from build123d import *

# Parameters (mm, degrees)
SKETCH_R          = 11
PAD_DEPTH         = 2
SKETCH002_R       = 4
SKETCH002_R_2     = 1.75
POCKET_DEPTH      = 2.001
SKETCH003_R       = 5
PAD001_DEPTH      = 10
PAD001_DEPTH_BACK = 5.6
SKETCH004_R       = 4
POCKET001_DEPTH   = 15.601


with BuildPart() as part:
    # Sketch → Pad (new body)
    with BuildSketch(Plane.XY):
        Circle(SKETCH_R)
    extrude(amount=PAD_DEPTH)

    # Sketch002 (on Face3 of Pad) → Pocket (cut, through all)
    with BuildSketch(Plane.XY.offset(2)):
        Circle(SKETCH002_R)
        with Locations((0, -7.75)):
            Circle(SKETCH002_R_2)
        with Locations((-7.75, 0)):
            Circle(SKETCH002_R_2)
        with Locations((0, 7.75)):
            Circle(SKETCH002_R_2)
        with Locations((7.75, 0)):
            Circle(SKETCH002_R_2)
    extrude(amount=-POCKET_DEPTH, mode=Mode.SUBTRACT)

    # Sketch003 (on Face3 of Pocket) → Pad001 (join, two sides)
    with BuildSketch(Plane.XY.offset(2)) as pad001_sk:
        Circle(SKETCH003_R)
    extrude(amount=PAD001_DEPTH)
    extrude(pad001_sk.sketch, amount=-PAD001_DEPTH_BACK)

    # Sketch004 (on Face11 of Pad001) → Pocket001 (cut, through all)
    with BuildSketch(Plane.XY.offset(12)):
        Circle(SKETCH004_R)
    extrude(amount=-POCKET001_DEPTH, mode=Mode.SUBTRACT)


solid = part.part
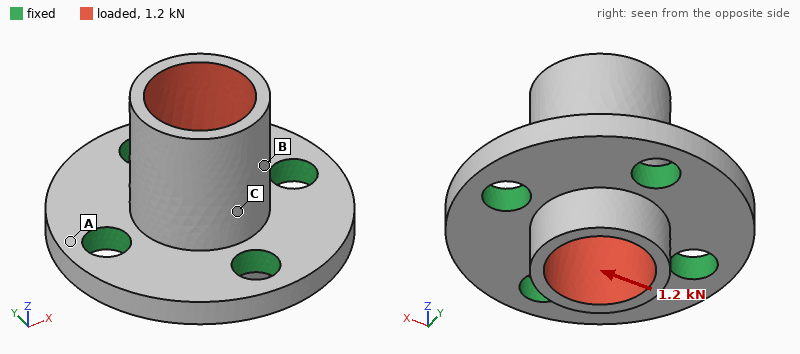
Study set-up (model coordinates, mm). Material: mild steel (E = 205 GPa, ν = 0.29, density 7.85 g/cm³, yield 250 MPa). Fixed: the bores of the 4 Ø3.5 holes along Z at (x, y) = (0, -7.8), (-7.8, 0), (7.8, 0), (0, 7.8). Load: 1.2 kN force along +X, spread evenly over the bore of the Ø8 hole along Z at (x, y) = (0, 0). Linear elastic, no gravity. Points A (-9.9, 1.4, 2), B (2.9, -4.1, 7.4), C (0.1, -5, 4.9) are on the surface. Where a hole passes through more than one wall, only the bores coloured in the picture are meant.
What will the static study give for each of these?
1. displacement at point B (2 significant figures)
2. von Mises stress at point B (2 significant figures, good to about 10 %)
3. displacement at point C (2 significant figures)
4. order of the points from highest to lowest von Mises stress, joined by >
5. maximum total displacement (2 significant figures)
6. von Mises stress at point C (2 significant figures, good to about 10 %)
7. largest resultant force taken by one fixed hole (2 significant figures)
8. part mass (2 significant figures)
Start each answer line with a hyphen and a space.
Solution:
- 5.1 µm
- 35 MPa
- 2.9 µm
- C > B > A
- 8.3 µm
- 53 MPa
- 440 N
- 7.6 g
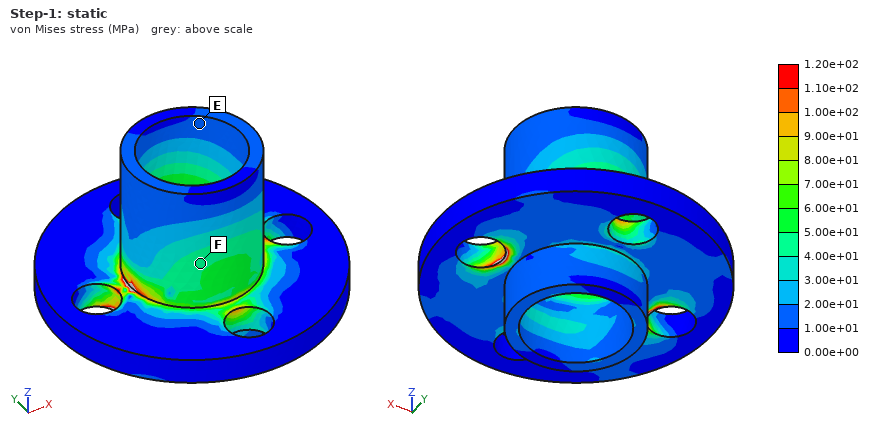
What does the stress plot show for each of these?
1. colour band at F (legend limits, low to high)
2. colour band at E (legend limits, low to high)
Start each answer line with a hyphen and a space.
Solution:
- 4.00e+01 to 5.00e+01 MPa
- 1.00e+01 to 2.00e+01 MPa
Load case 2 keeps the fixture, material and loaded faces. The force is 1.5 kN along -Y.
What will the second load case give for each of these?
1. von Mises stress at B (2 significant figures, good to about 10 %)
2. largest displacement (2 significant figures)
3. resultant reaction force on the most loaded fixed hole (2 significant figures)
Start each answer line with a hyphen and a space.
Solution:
- 35 MPa
- 10 µm
- 550 N
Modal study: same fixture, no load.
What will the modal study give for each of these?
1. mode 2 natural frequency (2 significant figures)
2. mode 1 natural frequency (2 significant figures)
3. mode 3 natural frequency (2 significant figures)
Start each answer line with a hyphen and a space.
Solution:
- 37 kHz
- 37 kHz
- 39 kHz
